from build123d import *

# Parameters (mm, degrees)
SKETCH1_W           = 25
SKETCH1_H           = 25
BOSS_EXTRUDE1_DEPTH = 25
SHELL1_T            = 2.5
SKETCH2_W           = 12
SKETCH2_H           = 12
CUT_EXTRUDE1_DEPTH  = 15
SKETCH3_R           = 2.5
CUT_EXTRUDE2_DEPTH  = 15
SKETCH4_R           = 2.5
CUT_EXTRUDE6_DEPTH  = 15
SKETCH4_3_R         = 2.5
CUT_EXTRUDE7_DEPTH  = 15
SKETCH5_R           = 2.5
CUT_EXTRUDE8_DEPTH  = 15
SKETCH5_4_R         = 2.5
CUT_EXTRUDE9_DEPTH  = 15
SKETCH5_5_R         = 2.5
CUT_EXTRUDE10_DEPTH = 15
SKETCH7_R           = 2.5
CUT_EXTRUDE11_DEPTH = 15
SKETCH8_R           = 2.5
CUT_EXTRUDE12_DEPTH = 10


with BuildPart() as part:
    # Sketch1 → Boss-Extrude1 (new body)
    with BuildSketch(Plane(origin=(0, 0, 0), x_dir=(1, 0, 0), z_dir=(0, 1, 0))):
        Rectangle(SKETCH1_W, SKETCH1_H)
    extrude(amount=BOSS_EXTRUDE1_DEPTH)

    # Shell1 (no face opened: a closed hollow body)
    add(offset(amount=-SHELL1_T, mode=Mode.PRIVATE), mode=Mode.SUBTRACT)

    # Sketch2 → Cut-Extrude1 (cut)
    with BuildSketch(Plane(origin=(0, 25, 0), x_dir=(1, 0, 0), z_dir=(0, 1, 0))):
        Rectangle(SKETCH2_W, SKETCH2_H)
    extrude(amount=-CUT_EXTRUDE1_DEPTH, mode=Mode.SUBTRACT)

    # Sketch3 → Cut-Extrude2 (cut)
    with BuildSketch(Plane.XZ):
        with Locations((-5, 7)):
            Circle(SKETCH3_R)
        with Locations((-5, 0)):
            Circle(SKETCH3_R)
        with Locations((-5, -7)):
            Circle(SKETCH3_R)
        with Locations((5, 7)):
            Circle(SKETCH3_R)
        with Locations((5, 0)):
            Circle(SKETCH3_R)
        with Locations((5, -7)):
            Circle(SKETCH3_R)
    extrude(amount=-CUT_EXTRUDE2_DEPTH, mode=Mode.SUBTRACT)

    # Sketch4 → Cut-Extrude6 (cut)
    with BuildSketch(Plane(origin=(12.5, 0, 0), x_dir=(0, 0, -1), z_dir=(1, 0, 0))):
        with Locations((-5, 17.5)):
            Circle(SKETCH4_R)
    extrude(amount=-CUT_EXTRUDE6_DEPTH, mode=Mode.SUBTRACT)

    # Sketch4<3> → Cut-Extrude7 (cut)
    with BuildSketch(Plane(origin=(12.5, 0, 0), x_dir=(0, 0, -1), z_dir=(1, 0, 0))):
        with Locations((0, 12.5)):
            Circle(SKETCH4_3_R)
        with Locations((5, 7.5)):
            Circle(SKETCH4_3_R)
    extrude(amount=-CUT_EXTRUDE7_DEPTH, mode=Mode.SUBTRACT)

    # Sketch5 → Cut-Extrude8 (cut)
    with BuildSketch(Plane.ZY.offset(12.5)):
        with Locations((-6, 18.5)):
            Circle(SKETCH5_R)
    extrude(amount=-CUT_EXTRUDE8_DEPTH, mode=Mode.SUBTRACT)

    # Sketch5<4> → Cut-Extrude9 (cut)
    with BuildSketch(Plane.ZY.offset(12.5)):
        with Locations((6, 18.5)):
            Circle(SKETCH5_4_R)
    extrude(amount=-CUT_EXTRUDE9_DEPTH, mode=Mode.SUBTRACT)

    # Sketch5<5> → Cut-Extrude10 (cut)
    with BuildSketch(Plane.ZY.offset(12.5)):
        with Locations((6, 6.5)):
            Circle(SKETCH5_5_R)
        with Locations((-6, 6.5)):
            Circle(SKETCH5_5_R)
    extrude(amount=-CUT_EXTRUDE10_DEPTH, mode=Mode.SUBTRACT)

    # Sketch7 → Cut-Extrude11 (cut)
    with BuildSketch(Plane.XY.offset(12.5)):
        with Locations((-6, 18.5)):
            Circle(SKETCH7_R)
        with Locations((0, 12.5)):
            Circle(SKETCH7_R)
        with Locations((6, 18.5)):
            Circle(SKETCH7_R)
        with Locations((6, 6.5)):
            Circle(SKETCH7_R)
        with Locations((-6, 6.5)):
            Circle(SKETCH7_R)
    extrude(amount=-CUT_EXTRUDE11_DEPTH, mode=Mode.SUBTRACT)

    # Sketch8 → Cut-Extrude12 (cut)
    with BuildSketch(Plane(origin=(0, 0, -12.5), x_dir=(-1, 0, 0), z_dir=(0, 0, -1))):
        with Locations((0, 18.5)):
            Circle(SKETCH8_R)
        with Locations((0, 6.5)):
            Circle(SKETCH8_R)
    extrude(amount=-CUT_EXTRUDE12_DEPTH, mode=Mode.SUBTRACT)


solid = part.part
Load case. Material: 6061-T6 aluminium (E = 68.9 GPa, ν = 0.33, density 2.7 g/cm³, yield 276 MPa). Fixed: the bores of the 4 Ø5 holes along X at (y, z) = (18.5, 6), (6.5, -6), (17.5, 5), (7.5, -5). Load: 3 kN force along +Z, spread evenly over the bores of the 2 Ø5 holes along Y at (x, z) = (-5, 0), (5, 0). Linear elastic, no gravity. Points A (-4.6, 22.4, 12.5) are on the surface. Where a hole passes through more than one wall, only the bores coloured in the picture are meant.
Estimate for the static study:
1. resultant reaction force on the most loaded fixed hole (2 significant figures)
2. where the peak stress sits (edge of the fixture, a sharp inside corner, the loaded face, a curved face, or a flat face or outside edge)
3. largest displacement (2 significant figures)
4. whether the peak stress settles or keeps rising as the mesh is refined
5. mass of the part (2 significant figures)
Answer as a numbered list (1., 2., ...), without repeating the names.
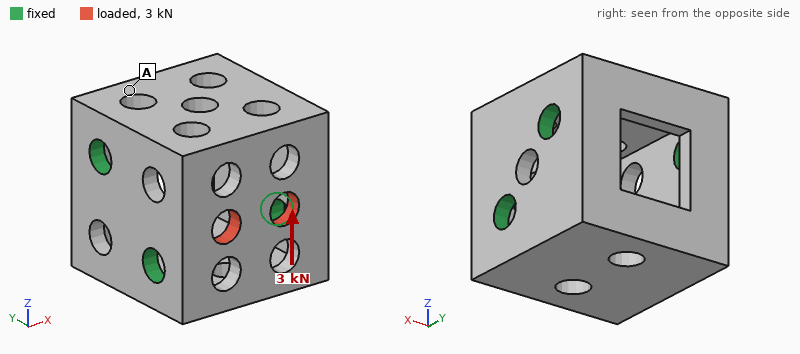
1. 1.6 kN
2. edge of the fixture
3. 26 µm
4. keeps rising
5. 17 g
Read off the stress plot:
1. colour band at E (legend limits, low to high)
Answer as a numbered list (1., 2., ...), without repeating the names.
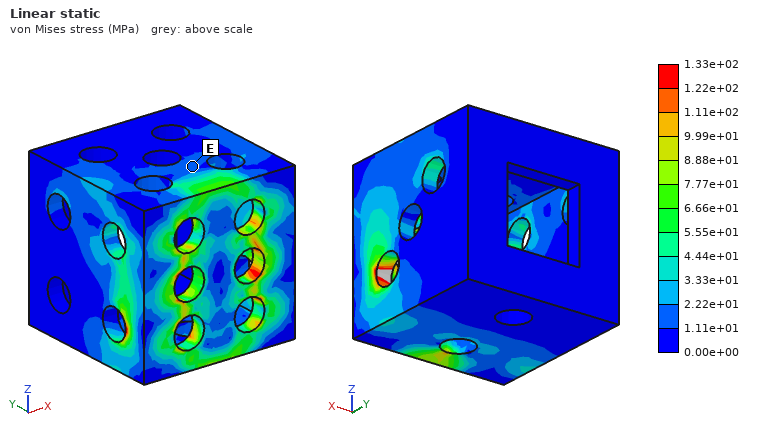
1. 1.11e+01 to 2.22e+01 MPa
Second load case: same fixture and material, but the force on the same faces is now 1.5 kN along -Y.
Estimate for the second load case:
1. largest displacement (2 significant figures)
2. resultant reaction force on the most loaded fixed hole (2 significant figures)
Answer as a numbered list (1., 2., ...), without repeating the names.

1. 56 µm
2. 540 N
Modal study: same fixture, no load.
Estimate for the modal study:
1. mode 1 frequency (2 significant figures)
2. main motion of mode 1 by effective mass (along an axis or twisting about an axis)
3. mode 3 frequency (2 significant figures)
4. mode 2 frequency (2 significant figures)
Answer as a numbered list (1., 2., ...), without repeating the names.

1. 23 kHz
2. along X
3. 26 kHz
4. 25 kHz
